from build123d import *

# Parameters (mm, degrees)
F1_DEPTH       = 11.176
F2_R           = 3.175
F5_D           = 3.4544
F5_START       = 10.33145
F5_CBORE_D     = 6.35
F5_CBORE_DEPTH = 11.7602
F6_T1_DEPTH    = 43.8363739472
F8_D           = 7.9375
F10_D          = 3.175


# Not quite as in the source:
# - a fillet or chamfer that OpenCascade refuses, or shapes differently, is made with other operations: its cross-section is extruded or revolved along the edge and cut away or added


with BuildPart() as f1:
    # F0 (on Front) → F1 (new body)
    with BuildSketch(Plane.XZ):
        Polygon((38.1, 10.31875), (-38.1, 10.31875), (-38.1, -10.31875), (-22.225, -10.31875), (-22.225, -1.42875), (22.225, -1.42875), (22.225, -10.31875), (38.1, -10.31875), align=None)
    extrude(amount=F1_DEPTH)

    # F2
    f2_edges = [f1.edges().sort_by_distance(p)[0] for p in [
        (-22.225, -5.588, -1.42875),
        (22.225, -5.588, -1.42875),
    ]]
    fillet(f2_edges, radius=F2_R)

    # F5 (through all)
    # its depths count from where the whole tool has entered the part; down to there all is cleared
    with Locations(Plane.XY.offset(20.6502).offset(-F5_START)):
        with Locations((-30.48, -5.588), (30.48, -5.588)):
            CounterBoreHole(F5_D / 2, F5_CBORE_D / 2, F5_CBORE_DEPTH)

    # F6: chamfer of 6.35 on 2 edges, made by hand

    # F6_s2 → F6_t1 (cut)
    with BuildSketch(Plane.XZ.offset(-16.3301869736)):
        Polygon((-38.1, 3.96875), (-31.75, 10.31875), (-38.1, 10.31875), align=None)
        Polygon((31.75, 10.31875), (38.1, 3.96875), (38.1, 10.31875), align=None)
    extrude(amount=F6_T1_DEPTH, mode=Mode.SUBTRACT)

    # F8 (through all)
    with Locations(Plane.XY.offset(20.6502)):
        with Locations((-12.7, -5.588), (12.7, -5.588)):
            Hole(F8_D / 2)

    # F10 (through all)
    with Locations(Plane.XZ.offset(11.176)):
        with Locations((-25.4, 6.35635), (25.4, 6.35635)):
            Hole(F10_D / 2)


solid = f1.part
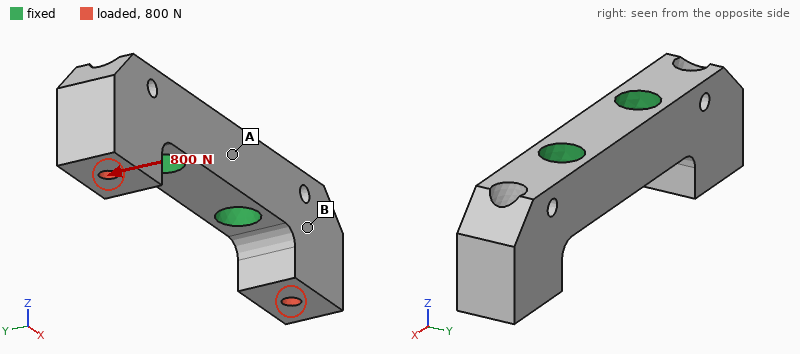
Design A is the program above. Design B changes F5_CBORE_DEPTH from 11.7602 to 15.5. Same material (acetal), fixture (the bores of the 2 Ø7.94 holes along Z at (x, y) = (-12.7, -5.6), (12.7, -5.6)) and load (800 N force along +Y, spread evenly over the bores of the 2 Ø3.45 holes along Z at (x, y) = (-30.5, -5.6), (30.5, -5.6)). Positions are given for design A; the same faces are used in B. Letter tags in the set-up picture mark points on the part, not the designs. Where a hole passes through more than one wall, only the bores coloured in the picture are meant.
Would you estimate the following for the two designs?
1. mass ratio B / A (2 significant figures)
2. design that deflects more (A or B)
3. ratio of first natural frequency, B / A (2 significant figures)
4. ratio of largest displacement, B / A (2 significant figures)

0.98
B
1.0
1.1
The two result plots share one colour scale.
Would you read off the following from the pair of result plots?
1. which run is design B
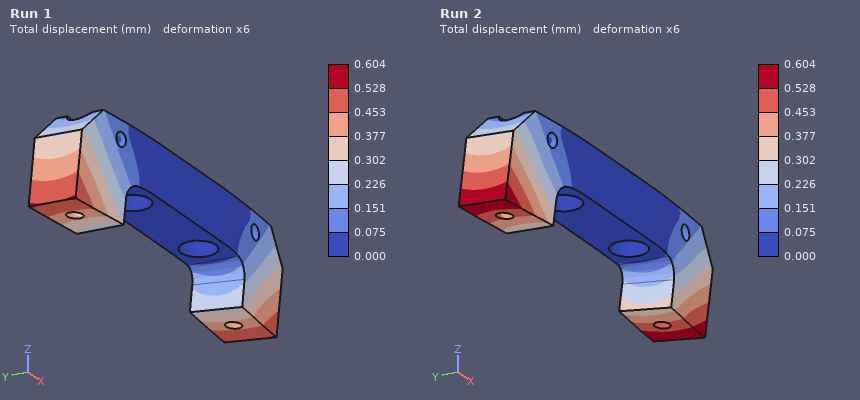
Run 2
